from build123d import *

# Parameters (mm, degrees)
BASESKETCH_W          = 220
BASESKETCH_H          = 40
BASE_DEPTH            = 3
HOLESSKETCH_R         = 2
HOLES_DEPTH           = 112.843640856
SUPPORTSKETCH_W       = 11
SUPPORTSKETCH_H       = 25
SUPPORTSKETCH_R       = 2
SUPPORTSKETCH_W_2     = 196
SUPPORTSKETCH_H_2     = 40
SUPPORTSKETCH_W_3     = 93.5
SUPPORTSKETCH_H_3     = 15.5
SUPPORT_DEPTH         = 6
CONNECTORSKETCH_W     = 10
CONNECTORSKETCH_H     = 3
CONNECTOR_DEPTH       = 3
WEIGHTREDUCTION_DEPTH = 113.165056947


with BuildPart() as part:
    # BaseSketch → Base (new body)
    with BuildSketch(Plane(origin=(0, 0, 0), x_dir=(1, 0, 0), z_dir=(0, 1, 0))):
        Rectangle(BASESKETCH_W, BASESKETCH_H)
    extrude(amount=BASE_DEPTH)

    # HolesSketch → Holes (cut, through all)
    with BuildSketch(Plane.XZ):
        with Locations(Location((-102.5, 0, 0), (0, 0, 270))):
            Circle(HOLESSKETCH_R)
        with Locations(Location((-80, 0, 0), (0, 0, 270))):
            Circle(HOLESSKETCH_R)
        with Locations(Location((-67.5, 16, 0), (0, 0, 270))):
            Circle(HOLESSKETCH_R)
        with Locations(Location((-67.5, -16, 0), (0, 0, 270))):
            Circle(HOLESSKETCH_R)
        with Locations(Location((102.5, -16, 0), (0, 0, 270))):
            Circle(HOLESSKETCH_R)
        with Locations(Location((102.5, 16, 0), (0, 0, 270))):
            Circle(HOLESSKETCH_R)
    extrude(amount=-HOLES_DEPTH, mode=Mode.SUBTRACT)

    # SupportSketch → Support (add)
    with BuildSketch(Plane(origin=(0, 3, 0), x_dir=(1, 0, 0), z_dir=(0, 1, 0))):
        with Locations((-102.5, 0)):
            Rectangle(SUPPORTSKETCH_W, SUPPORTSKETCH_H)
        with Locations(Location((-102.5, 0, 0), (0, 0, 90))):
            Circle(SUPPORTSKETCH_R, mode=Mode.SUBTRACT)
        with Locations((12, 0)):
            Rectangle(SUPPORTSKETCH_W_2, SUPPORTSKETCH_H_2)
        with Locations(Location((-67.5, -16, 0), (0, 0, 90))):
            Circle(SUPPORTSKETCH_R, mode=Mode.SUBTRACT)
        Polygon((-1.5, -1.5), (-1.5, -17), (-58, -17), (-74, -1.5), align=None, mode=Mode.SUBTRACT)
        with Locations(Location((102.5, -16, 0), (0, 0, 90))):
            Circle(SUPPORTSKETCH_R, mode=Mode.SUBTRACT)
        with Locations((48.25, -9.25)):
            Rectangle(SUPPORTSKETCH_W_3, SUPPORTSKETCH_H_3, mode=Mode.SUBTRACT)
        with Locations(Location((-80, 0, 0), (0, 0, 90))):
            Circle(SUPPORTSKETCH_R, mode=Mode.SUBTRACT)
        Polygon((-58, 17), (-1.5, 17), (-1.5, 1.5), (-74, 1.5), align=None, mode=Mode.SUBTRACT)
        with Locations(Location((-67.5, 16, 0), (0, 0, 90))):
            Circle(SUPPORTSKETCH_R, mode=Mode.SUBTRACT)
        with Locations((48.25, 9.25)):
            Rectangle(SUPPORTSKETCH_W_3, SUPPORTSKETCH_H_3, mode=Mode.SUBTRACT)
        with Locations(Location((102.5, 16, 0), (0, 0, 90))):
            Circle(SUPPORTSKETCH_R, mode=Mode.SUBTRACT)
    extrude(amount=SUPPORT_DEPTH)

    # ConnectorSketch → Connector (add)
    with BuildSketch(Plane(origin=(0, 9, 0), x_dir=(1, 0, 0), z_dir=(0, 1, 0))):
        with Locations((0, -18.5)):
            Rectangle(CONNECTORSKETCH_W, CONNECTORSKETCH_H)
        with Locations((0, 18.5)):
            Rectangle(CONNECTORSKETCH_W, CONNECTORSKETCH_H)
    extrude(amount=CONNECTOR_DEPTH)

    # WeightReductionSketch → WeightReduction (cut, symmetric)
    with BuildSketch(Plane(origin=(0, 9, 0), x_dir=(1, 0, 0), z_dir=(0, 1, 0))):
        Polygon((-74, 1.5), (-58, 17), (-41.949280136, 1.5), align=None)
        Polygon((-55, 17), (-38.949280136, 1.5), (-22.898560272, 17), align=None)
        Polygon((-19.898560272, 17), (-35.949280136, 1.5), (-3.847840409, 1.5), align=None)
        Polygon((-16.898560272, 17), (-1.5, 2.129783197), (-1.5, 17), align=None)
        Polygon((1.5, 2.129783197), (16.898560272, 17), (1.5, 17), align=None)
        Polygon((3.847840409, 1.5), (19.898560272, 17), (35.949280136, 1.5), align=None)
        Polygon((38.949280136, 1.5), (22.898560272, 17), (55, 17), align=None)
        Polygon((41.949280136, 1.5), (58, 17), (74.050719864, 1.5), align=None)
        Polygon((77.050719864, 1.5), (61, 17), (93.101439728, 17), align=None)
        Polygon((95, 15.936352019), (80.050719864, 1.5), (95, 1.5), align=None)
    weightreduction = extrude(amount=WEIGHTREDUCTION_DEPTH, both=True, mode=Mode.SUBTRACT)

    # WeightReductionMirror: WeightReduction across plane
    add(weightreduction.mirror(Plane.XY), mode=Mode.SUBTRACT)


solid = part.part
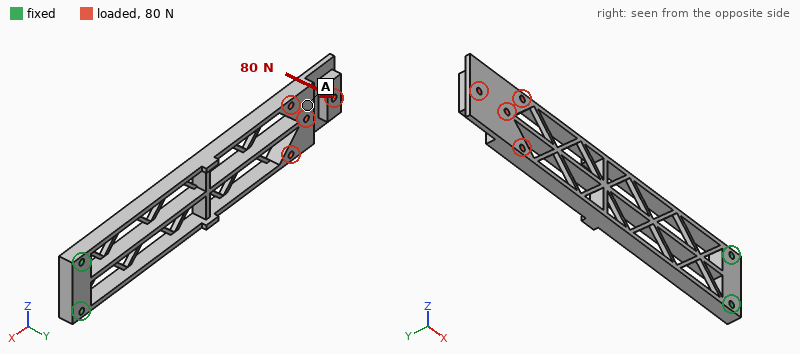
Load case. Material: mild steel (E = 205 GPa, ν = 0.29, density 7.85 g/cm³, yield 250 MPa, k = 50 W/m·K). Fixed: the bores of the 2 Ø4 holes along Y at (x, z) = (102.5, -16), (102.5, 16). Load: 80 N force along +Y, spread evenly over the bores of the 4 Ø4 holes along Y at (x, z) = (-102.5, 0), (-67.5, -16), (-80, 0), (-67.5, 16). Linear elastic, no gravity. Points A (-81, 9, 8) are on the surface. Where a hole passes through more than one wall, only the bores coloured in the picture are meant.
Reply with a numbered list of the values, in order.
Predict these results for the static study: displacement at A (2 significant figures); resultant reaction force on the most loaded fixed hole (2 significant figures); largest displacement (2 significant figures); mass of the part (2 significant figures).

1. 1.3 mm
2. 68 N
3. 1.6 mm
4. 260 g
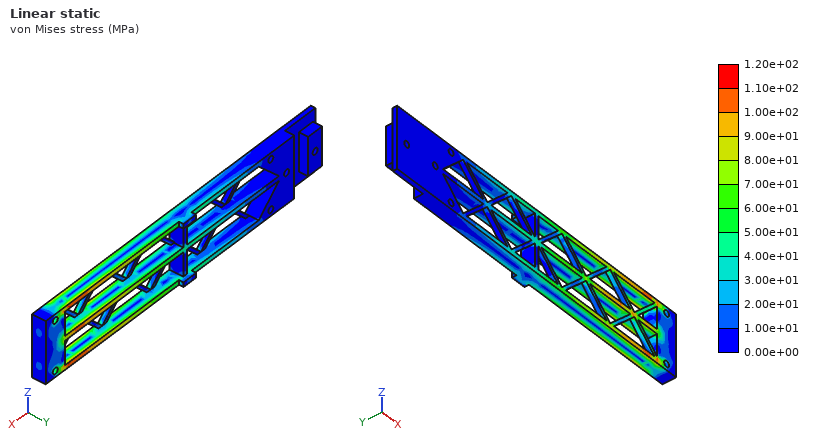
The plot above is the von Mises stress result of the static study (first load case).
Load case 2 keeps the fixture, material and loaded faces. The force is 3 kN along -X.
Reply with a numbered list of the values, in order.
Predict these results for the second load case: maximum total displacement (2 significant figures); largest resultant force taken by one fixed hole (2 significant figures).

1. 67 µm
2. 1.5 kN
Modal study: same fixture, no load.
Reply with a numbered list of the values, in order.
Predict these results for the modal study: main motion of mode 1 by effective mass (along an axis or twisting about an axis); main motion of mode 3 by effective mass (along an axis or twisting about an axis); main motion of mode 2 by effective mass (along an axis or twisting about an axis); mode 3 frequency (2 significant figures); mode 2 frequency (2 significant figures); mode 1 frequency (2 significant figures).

1. along Y
2. along Z
3. along Z
4. 640 Hz
5. 420 Hz
6. 110 Hz
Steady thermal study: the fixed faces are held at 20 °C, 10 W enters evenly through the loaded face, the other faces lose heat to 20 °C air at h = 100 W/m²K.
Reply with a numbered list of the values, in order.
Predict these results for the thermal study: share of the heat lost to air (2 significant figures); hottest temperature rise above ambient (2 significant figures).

1. 100 %
2. 16 K
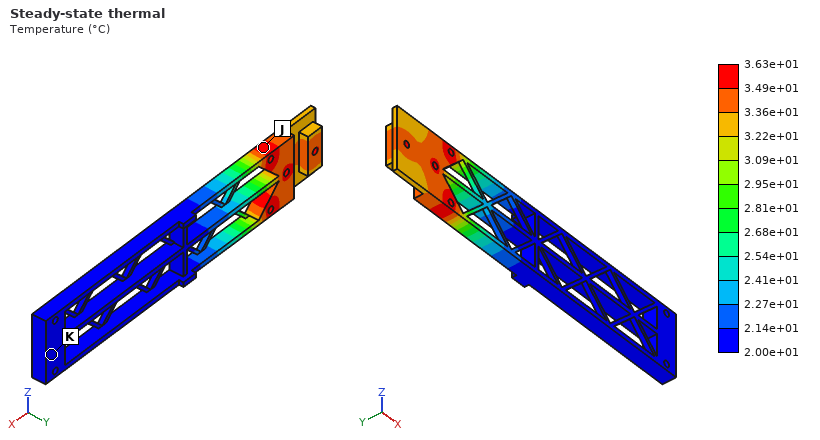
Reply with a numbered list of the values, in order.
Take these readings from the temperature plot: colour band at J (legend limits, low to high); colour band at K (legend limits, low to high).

1. 3.49e+01 to 3.63e+01 °C
2. 2.00e+01 to 2.14e+01 °C
